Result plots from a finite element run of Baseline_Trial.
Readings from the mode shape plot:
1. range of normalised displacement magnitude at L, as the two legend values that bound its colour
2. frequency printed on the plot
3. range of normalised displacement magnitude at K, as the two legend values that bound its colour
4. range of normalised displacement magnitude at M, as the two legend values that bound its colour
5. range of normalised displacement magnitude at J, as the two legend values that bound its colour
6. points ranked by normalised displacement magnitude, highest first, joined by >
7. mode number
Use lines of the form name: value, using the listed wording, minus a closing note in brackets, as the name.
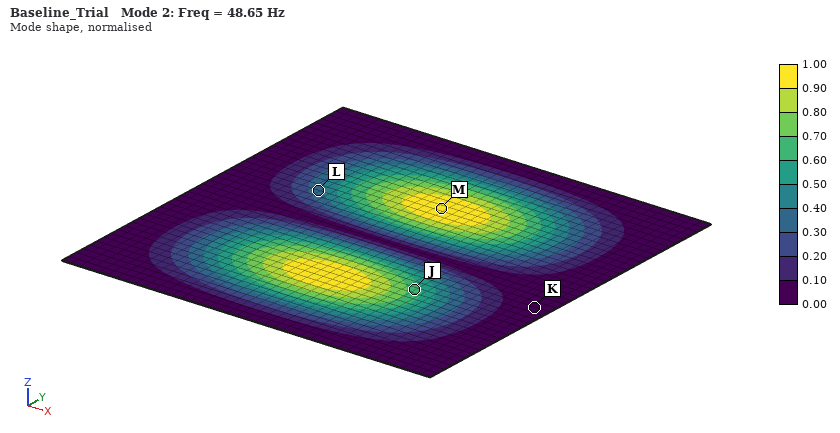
range of normalised displacement magnitude at L, as the two legend values that bound its colour: 0.30 to 0.40
frequency printed on the plot: 48.65 Hz
range of normalised displacement magnitude at K, as the two legend values that bound its colour: 0.00 to 0.10
range of normalised displacement magnitude at M, as the two legend values that bound its colour: 0.90 to 1.00
range of normalised displacement magnitude at J, as the two legend values that bound its colour: 0.60 to 0.70
points ranked by normalised displacement magnitude, highest first, joined by >: M > J > L > K
mode number: 2
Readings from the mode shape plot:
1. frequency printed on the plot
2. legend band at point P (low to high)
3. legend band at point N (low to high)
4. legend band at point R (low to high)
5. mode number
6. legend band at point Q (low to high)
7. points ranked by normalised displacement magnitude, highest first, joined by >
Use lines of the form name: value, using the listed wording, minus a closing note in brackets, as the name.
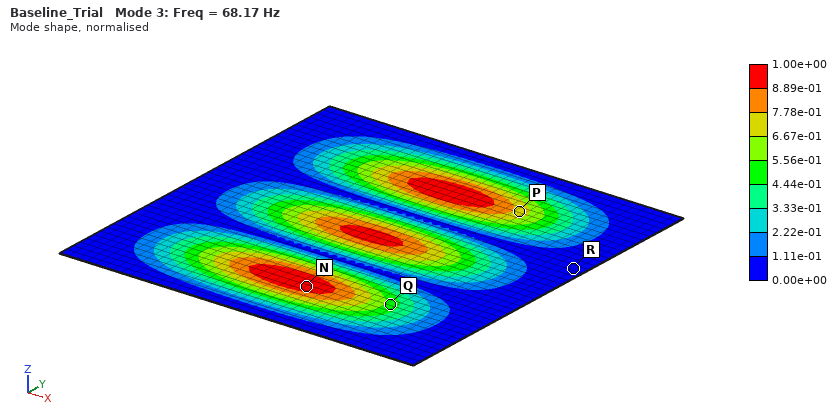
frequency printed on the plot: 68.17 Hz
legend band at point P: 6.67e-01 to 7.78e-01
legend band at point N: 8.89e-01 to 1.00e+00
legend band at point R: 0.00e+00 to 1.11e-01
mode number: 3
legend band at point Q: 4.44e-01 to 5.56e-01
points ranked by normalised displacement magnitude, highest first, joined by >: N > P > Q > R
